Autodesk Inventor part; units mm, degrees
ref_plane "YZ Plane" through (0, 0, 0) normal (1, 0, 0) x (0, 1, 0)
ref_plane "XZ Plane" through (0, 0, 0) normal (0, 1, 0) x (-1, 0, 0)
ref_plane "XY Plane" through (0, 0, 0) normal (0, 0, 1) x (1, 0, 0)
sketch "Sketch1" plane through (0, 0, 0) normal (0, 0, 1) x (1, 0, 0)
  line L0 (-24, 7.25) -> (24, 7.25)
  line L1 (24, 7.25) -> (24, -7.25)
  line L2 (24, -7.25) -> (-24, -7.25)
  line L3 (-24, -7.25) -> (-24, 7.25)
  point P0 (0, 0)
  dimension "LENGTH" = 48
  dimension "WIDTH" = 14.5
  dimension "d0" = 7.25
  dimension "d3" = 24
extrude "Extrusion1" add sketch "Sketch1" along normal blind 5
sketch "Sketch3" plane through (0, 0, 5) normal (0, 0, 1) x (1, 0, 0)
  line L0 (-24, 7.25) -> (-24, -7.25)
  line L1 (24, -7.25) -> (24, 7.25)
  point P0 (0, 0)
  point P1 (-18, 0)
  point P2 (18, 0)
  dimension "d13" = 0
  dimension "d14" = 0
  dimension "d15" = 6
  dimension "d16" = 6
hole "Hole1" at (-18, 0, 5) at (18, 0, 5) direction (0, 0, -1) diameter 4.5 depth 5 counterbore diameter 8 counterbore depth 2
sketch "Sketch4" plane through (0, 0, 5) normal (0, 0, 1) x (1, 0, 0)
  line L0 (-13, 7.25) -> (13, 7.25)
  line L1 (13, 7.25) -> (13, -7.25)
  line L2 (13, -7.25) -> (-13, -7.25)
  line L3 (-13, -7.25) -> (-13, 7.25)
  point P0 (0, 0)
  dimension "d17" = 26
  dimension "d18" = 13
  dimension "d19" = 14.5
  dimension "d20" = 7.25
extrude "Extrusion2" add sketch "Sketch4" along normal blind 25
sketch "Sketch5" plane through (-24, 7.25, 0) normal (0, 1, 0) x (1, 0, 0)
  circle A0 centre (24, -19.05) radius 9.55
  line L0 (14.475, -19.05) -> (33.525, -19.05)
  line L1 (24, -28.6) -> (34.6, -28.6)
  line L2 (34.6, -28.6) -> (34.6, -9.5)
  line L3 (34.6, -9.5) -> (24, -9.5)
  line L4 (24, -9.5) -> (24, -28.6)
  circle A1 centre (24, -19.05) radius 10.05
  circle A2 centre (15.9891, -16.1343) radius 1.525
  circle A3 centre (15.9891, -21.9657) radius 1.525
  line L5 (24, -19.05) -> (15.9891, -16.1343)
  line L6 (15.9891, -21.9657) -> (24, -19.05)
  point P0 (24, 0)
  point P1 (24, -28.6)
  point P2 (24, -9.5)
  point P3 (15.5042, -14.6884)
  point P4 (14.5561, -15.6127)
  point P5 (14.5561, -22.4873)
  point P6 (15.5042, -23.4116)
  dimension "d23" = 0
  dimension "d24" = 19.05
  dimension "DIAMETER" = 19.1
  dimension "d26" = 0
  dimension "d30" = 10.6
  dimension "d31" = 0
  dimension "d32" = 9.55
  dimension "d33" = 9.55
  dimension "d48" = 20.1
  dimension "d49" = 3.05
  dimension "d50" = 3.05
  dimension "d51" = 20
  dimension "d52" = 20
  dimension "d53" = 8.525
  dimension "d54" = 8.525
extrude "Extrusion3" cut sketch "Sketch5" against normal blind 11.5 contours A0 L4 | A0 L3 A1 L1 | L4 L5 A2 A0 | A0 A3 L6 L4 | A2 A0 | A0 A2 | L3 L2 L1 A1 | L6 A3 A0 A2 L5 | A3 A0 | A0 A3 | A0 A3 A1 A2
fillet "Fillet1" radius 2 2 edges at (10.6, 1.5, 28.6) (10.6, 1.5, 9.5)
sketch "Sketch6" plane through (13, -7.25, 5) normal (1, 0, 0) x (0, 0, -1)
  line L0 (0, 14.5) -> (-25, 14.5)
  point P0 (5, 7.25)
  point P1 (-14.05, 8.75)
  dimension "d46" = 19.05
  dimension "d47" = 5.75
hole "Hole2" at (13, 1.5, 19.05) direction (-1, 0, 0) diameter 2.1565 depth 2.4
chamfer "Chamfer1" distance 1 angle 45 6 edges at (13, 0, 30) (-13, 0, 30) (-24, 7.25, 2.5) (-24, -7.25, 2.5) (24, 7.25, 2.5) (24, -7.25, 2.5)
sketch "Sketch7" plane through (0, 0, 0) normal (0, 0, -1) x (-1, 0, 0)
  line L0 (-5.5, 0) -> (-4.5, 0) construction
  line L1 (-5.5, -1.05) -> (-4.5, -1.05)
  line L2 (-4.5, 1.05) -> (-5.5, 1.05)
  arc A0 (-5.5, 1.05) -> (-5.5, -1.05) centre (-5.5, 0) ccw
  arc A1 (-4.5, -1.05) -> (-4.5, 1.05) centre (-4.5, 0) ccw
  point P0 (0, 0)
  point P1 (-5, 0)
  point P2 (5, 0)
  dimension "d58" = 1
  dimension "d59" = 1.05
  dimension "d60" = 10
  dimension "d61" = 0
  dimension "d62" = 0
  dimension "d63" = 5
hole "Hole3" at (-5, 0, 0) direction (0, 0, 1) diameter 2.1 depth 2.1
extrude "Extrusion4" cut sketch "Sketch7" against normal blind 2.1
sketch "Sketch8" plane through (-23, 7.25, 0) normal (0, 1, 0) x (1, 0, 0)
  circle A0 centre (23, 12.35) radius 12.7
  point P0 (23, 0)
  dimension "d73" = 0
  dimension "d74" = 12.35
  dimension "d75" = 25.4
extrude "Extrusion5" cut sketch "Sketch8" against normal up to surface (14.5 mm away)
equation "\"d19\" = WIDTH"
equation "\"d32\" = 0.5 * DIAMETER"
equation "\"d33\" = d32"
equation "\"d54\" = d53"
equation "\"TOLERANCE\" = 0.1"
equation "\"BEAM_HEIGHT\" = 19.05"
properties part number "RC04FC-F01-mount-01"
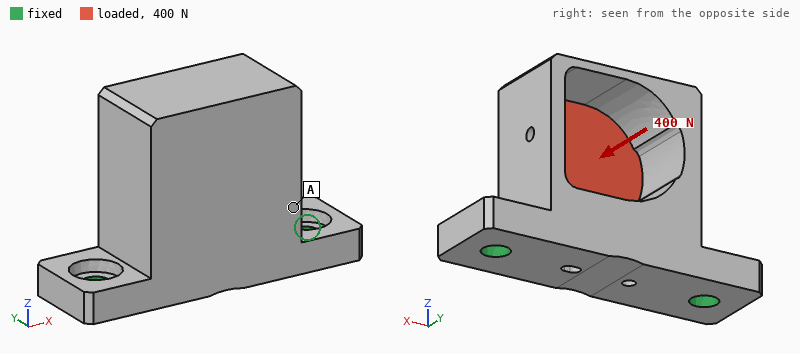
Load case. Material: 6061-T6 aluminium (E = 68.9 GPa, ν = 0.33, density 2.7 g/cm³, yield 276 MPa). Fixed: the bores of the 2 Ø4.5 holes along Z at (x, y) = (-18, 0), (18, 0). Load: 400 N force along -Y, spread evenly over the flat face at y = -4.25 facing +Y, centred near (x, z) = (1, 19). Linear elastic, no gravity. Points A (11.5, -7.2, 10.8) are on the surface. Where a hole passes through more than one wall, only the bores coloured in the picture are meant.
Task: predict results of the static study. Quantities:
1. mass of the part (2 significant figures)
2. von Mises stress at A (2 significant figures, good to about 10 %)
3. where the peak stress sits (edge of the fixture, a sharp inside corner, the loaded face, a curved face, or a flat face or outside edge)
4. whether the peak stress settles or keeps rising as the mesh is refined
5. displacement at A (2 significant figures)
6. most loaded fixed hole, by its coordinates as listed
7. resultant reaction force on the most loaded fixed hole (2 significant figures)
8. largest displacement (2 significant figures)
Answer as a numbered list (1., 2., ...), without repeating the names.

1. 23 g
2. 13 MPa
3. edge of the fixture
4. keeps rising
5. 29 µm
6. (18, 0)
7. 210 N
8. 76 µm
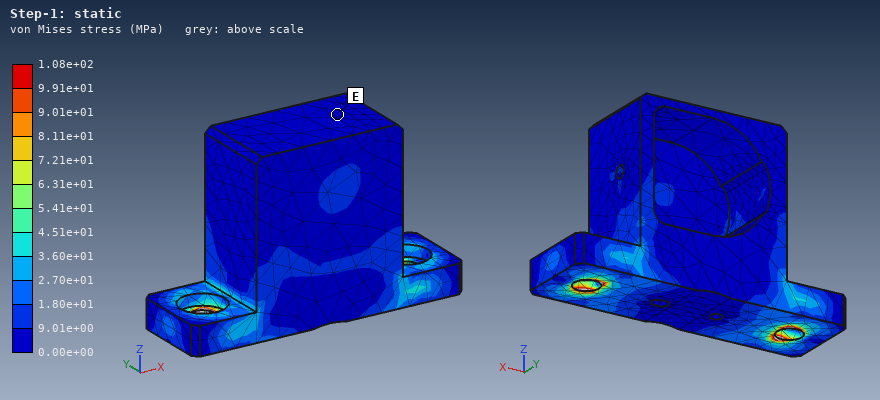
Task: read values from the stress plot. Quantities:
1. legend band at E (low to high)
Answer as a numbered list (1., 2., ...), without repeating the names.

1. 0.00e+00 to 9.01e+00 MPa
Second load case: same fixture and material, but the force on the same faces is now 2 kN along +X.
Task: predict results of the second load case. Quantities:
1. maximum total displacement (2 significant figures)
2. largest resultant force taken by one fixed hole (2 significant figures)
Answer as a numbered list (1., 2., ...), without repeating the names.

1. 54 µm
2. 1.6 kN
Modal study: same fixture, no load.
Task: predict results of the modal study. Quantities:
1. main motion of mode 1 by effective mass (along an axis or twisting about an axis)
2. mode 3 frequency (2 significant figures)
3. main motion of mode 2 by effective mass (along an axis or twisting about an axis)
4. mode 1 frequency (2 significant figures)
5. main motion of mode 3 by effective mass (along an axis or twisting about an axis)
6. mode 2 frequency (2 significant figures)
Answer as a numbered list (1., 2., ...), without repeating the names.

1. along Y
2. 15 kHz
3. along X
4. 3900 Hz
5. along Z
6. 9400 Hz
